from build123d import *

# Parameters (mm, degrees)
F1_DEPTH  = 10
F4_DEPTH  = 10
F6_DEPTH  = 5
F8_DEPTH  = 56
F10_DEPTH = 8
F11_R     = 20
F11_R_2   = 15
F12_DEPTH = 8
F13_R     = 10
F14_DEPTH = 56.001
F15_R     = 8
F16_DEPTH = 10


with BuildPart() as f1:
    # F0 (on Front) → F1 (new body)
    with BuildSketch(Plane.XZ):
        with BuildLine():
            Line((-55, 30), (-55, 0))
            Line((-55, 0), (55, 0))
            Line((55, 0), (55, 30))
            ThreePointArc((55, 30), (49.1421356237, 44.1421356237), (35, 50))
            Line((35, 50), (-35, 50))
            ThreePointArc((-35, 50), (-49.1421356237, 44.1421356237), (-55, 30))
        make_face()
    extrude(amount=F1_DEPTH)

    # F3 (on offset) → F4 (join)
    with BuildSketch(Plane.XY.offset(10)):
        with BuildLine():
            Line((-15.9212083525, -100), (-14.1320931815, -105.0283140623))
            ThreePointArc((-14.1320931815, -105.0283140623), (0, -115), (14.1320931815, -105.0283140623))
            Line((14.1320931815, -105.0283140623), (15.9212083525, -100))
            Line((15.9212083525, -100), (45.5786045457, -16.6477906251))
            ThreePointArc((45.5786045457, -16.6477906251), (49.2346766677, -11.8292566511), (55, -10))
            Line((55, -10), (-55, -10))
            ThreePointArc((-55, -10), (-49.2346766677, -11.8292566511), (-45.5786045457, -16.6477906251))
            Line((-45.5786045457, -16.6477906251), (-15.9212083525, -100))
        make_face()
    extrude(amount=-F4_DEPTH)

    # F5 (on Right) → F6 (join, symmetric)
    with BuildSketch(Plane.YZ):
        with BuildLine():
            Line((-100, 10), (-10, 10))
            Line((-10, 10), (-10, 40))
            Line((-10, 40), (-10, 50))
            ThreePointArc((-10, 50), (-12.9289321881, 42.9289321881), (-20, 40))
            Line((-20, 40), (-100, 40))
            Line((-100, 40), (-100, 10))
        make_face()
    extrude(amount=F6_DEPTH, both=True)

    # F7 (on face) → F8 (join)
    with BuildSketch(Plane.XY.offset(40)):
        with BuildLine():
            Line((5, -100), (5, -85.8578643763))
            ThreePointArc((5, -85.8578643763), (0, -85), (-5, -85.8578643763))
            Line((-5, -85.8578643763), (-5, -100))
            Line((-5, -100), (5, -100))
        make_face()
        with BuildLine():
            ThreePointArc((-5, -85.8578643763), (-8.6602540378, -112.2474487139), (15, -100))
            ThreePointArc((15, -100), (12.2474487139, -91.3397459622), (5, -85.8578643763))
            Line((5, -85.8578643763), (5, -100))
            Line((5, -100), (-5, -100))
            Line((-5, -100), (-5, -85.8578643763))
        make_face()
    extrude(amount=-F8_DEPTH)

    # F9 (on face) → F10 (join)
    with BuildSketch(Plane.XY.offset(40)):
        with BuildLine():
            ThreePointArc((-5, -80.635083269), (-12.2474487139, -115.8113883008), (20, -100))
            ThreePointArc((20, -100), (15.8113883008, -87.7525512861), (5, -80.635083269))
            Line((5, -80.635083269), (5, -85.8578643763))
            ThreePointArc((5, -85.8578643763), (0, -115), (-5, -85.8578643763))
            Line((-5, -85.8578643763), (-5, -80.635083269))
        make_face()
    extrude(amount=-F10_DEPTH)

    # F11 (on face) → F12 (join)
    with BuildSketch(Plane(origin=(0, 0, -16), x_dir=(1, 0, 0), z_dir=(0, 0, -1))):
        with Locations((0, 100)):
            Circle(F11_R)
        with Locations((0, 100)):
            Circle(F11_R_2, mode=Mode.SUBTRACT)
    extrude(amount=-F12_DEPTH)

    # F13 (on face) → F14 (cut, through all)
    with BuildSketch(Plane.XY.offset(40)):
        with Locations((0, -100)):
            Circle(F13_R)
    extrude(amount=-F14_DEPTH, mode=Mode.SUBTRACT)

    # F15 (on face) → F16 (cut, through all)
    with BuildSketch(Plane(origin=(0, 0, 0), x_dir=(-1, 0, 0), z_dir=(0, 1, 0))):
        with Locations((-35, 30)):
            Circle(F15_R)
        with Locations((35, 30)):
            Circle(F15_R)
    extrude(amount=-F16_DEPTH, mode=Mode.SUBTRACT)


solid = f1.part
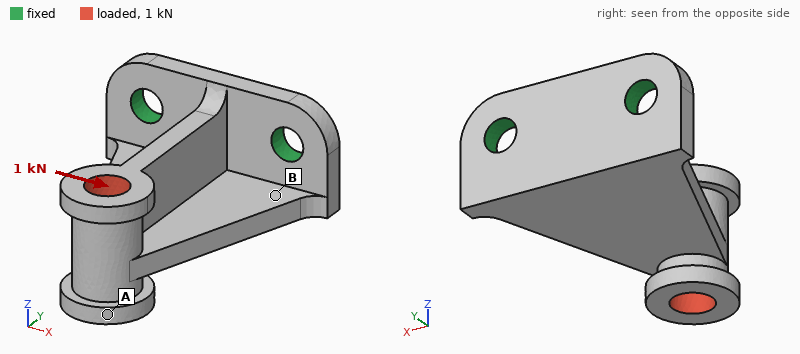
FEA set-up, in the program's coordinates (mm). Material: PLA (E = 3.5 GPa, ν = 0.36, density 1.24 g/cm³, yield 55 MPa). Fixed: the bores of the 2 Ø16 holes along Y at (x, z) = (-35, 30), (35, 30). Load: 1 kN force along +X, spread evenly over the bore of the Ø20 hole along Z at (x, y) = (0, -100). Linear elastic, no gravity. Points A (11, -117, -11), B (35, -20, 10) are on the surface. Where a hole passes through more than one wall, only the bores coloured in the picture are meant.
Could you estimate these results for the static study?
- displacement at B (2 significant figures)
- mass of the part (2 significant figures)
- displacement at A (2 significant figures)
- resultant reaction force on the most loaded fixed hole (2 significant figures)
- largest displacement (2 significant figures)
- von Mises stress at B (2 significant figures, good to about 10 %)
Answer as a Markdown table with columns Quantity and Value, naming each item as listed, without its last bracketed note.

| Quantity | Value |
|---|---|
| displacement at B | 0.25 mm |
| mass of the part | 190 g |
| displacement at A | 0.90 mm |
| resultant reaction force on the most loaded fixed hole | 1.5 kN |
| largest displacement | 1.6 mm |
| von Mises stress at B | 12 MPa |
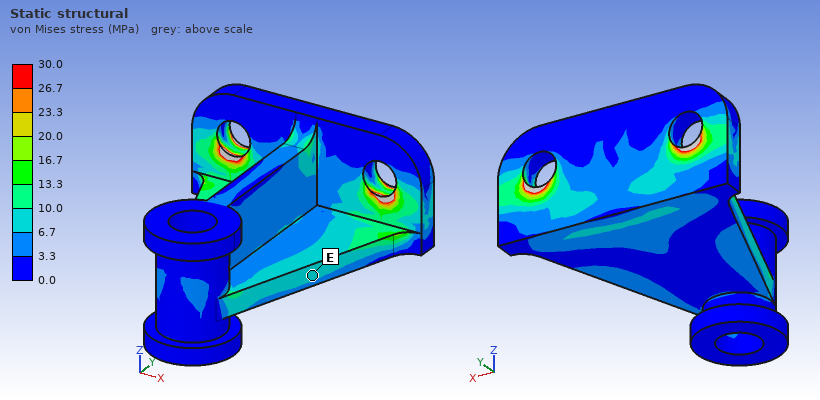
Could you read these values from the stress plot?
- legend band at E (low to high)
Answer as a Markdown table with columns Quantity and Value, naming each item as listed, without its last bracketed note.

| Quantity | Value |
|---|---|
| legend band at E | 6.7 to 10.0 MPa |
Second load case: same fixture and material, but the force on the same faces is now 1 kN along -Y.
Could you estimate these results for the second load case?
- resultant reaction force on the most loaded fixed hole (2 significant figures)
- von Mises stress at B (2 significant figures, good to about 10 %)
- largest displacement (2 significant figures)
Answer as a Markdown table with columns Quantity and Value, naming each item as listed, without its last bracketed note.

| Quantity | Value |
|---|---|
| resultant reaction force on the most loaded fixed hole | 510 N |
| von Mises stress at B | 2.8 MPa |
| largest displacement | 0.35 mm |
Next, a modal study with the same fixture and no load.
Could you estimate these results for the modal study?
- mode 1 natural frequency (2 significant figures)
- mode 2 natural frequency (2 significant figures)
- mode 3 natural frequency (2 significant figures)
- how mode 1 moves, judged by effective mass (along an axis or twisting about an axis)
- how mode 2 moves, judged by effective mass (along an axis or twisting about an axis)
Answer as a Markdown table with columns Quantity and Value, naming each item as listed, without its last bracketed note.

| Quantity | Value |
|---|---|
| mode 1 natural frequency | 350 Hz |
| mode 2 natural frequency | 610 Hz |
| mode 3 natural frequency | 950 Hz |
| how mode 1 moves, judged by effective mass | along Z |
| how mode 2 moves, judged by effective mass | along X |
